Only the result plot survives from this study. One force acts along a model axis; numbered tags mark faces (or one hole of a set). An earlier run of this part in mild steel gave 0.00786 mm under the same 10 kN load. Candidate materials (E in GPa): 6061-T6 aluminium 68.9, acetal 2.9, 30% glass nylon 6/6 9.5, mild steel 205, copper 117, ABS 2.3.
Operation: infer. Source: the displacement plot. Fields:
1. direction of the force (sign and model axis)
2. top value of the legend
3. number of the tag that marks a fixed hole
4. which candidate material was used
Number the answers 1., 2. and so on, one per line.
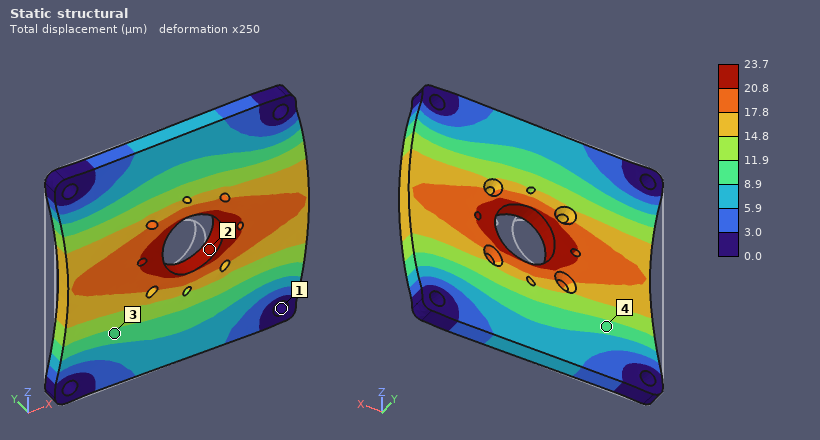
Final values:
1. +X
2. 23.7 µm
3. 1
4. 6061-T6 aluminium
